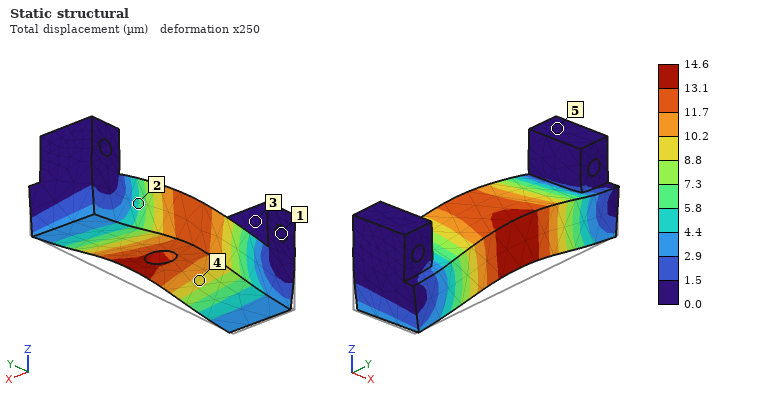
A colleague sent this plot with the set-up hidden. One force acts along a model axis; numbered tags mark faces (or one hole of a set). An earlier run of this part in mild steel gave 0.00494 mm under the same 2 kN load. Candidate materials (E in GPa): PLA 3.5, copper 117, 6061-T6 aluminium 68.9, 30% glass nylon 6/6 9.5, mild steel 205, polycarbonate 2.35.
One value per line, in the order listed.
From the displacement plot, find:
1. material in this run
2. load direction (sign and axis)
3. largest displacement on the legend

6061-T6 aluminium
+Z
14.6 µm
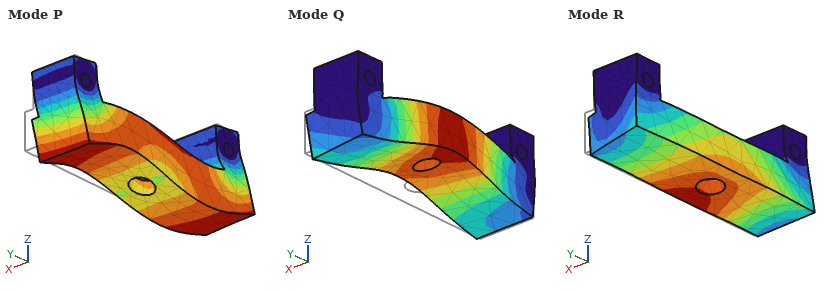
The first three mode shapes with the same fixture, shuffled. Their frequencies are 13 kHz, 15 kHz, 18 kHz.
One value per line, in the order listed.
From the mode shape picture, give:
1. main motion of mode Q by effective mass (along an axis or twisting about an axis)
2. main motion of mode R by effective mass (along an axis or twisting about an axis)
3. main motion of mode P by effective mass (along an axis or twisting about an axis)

along Z
along X
along Y
